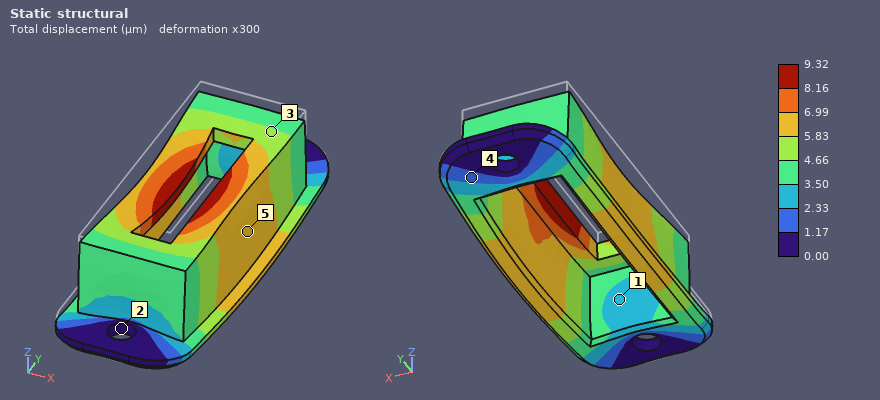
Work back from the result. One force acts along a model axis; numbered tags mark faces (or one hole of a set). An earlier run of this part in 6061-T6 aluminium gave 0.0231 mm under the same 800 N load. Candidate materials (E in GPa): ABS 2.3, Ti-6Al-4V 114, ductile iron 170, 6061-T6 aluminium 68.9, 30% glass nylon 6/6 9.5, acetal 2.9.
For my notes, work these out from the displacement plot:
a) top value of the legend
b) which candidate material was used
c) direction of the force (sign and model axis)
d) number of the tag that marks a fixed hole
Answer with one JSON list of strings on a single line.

["9.32 µm", "ductile iron", "-Z", "2"]
